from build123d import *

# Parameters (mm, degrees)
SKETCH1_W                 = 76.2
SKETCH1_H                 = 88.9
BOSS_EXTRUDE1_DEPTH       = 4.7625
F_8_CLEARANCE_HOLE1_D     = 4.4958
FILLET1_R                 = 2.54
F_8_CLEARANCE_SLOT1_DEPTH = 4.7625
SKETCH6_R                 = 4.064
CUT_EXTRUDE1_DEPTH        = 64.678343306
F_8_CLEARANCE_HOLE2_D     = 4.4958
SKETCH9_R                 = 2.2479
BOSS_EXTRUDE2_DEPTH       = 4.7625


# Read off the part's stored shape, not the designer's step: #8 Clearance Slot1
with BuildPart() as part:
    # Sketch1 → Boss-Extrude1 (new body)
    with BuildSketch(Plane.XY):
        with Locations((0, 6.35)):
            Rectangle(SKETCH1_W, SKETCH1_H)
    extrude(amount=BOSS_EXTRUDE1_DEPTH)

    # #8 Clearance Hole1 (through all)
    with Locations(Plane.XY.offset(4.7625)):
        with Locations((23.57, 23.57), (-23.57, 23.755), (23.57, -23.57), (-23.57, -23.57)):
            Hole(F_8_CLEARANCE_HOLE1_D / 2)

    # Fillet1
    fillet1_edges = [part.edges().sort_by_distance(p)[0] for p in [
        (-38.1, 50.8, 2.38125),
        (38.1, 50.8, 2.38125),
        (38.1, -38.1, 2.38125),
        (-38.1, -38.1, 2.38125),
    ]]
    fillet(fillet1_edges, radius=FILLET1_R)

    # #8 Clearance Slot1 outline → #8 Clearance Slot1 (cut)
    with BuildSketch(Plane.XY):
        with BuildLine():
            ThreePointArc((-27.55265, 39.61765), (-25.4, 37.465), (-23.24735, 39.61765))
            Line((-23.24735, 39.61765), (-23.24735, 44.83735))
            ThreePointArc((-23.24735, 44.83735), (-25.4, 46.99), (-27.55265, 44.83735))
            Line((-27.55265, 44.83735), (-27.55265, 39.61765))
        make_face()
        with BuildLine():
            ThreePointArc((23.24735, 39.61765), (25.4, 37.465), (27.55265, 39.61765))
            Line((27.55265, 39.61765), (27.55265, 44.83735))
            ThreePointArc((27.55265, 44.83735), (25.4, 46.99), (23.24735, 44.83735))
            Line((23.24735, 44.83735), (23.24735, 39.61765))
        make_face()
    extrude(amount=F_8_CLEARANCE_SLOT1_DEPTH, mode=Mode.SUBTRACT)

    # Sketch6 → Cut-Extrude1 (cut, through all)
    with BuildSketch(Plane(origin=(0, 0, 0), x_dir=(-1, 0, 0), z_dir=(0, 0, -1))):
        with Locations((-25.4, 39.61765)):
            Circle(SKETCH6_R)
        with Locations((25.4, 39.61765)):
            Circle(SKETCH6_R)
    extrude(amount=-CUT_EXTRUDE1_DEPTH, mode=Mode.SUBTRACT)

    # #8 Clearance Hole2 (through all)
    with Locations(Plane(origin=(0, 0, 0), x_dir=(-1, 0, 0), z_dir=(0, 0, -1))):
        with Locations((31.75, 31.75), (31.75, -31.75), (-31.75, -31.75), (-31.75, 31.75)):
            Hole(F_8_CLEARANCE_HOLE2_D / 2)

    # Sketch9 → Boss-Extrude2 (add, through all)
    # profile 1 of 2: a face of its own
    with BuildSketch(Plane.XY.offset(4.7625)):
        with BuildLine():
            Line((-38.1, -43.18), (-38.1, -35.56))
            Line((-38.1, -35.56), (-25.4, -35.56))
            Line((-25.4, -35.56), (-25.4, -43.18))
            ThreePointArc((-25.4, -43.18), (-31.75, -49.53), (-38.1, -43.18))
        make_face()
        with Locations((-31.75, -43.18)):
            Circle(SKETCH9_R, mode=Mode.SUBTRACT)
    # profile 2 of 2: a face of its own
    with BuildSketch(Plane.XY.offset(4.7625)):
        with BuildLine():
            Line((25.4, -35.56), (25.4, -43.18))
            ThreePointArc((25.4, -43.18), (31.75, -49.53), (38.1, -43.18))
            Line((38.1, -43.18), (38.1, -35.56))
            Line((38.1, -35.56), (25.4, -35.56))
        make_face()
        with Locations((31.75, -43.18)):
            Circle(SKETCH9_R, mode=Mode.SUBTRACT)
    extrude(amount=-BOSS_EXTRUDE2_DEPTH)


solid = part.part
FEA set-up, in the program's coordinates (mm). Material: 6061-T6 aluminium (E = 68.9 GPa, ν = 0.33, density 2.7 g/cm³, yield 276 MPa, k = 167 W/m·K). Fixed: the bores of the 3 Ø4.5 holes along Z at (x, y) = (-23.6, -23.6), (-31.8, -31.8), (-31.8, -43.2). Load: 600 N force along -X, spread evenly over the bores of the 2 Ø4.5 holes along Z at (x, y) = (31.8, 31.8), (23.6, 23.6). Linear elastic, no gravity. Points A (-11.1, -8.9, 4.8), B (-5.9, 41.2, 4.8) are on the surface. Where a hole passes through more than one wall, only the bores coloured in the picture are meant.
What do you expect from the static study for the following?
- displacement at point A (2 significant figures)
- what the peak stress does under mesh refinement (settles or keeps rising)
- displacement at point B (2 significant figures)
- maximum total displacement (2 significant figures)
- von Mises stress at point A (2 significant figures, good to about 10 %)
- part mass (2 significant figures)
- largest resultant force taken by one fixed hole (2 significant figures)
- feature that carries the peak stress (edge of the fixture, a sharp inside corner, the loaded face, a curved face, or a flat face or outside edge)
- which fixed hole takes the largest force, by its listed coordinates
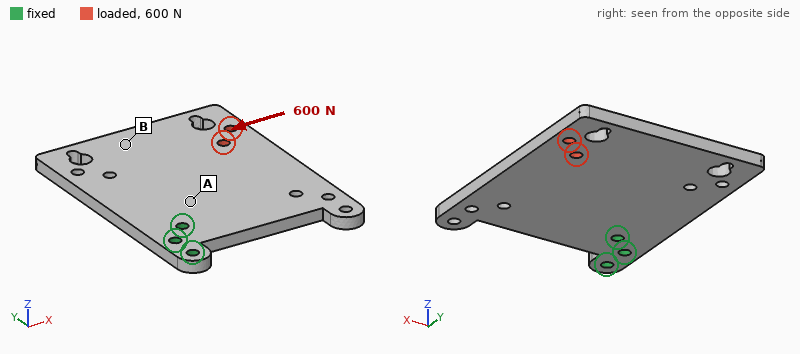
0.022 mm
keeps rising
0.077 mm
0.11 mm
8.0 MPa
87 g
2.2 kN
edge of the fixture
(-23.6, -23.6)
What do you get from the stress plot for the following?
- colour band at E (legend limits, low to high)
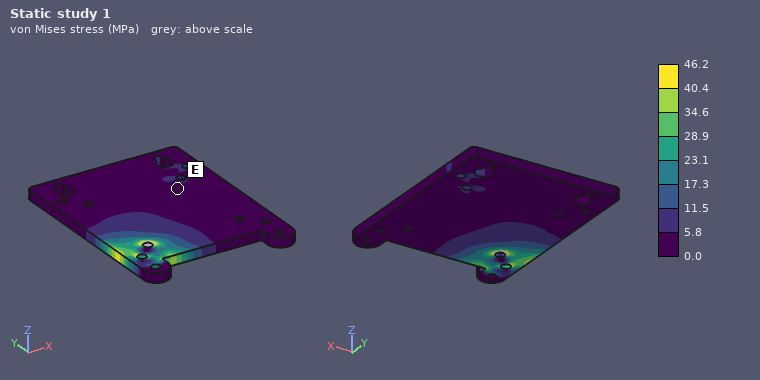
0.0 to 5.8 MPa
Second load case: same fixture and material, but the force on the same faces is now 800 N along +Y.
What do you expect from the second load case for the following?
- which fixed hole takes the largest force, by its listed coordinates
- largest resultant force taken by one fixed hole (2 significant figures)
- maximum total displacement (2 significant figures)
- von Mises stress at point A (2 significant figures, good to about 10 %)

(-23.6, -23.6)
2.8 kN
0.14 mm
10 MPa
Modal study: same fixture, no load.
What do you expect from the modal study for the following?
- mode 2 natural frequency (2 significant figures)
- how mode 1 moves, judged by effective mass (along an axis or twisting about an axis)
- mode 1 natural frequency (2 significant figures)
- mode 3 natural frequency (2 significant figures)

840 Hz
along Z
490 Hz
1800 Hz
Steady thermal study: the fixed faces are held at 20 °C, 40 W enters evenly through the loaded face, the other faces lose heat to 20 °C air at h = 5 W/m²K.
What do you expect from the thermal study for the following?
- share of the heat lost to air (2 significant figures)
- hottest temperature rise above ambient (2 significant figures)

7.4 %
79 K
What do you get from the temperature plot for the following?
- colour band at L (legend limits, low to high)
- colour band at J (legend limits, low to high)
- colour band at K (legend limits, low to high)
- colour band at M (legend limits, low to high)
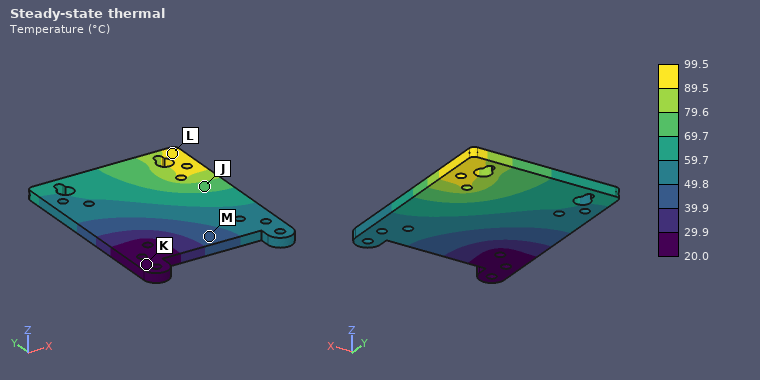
89.5 to 99.5 °C
69.7 to 79.6 °C
20.0 to 29.9 °C
39.9 to 49.8 °C
